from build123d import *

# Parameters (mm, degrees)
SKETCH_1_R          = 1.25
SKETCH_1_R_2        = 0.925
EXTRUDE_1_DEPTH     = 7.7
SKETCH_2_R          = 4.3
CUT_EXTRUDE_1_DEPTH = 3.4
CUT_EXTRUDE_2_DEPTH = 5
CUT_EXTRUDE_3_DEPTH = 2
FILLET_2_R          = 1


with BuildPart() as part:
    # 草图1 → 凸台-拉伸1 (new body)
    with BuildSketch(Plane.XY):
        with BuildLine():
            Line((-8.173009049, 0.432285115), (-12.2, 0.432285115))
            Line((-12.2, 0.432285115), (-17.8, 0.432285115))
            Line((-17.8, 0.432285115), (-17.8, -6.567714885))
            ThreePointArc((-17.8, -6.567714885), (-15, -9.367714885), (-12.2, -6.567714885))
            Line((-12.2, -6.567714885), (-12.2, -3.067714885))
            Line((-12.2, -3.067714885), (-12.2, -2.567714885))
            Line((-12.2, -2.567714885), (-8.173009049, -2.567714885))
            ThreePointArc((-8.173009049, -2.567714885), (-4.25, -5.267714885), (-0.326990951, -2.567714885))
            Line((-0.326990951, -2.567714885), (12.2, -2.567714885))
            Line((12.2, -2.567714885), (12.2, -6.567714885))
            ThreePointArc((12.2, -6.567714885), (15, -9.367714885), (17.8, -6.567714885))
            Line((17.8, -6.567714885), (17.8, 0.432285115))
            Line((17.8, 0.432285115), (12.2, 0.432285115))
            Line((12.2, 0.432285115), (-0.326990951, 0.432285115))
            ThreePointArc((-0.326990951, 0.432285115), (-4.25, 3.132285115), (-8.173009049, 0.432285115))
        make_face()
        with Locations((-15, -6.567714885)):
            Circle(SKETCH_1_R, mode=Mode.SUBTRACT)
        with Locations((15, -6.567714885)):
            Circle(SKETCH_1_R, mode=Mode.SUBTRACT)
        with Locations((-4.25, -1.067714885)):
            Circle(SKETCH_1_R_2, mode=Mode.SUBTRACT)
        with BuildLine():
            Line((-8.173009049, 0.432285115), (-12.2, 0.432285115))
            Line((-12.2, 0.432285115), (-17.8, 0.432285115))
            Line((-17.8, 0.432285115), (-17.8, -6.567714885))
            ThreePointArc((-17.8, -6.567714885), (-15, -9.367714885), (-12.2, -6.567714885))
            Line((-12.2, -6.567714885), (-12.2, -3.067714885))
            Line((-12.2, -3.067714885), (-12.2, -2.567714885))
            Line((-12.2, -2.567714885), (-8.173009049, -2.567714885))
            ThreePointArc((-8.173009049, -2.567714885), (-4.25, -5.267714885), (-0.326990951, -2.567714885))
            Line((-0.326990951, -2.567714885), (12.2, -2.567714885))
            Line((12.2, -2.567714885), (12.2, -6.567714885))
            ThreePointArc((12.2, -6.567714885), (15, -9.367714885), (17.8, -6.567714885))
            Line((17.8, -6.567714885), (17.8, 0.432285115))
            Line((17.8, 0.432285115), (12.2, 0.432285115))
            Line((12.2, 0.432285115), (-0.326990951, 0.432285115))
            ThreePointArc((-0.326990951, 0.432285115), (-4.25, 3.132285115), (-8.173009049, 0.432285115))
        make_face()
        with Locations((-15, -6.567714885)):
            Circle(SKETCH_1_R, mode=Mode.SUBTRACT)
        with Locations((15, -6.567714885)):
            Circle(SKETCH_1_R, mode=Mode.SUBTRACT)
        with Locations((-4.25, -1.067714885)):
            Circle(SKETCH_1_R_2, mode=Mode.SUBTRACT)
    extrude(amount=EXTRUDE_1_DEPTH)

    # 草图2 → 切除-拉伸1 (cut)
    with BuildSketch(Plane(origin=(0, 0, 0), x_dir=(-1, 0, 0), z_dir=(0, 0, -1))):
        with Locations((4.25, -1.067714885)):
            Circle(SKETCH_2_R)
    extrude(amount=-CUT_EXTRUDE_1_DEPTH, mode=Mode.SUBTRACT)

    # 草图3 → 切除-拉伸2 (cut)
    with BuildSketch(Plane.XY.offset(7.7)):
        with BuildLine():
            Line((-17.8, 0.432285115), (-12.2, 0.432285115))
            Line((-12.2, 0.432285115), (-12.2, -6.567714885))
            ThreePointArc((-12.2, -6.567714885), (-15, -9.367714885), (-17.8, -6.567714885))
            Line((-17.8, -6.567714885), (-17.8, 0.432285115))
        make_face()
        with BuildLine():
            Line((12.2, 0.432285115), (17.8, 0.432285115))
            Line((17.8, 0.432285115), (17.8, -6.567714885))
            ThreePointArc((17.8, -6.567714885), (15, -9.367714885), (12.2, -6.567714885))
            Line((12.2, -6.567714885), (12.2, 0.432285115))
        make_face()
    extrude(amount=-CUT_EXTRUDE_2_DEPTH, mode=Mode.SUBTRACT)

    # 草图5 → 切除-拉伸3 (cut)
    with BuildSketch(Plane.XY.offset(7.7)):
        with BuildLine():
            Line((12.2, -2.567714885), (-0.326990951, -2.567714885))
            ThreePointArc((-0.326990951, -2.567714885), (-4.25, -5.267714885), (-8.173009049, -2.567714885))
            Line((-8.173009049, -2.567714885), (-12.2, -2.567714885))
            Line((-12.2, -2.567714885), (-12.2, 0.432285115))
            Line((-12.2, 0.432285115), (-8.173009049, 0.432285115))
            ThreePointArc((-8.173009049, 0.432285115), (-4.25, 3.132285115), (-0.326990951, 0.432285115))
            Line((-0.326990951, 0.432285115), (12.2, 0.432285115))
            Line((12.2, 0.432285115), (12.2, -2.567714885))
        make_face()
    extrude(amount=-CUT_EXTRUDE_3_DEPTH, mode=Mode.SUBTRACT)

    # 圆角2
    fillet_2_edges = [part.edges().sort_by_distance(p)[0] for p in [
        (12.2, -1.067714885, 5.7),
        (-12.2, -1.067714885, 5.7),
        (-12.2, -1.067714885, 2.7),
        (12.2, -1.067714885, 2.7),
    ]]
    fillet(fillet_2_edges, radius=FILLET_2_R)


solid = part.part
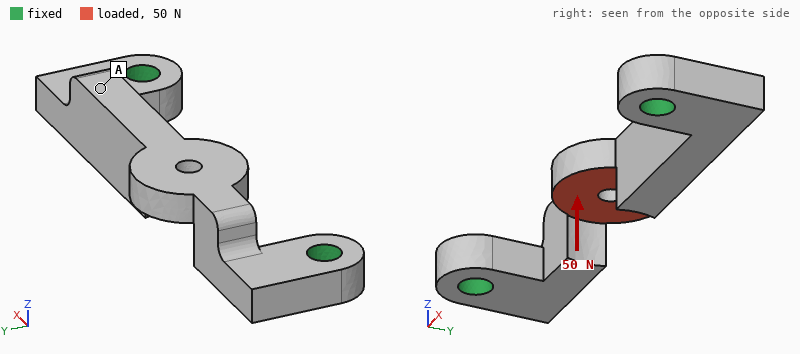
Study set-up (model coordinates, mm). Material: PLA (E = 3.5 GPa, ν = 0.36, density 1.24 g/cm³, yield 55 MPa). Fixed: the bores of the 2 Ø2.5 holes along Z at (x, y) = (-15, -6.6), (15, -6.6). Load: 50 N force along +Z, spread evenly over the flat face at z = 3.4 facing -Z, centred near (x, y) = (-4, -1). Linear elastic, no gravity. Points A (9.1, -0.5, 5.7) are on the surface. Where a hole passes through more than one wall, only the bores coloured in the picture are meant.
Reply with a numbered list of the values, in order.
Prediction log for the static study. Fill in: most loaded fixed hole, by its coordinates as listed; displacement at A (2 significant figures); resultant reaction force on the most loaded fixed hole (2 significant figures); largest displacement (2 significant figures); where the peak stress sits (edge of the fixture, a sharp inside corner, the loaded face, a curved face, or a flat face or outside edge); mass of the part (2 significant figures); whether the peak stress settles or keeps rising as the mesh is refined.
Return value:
1. (-15, -6.6)
2. 0.13 mm
3. 53 N
4. 0.31 mm
5. a sharp inside corner
6. 0.80 g
7. keeps rising
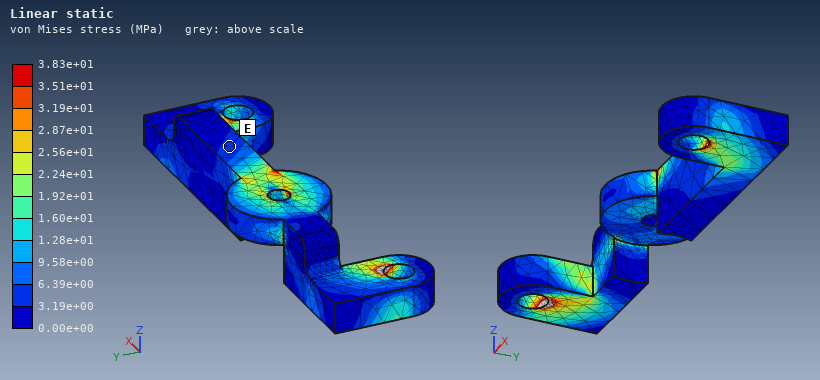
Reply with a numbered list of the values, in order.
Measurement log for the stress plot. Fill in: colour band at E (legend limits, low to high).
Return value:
1. 3.19e+00 to 6.39e+00 MPa
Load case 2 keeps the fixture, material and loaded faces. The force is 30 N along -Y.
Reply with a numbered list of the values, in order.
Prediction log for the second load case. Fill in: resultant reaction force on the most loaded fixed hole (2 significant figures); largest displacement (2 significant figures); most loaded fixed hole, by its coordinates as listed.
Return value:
1. 21 N
2. 0.15 mm
3. (-15, -6.6)
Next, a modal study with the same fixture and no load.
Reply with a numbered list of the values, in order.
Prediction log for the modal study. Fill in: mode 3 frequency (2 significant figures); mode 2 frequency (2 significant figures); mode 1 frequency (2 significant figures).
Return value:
1. 7500 Hz
2. 5200 Hz
3. 3500 Hz
